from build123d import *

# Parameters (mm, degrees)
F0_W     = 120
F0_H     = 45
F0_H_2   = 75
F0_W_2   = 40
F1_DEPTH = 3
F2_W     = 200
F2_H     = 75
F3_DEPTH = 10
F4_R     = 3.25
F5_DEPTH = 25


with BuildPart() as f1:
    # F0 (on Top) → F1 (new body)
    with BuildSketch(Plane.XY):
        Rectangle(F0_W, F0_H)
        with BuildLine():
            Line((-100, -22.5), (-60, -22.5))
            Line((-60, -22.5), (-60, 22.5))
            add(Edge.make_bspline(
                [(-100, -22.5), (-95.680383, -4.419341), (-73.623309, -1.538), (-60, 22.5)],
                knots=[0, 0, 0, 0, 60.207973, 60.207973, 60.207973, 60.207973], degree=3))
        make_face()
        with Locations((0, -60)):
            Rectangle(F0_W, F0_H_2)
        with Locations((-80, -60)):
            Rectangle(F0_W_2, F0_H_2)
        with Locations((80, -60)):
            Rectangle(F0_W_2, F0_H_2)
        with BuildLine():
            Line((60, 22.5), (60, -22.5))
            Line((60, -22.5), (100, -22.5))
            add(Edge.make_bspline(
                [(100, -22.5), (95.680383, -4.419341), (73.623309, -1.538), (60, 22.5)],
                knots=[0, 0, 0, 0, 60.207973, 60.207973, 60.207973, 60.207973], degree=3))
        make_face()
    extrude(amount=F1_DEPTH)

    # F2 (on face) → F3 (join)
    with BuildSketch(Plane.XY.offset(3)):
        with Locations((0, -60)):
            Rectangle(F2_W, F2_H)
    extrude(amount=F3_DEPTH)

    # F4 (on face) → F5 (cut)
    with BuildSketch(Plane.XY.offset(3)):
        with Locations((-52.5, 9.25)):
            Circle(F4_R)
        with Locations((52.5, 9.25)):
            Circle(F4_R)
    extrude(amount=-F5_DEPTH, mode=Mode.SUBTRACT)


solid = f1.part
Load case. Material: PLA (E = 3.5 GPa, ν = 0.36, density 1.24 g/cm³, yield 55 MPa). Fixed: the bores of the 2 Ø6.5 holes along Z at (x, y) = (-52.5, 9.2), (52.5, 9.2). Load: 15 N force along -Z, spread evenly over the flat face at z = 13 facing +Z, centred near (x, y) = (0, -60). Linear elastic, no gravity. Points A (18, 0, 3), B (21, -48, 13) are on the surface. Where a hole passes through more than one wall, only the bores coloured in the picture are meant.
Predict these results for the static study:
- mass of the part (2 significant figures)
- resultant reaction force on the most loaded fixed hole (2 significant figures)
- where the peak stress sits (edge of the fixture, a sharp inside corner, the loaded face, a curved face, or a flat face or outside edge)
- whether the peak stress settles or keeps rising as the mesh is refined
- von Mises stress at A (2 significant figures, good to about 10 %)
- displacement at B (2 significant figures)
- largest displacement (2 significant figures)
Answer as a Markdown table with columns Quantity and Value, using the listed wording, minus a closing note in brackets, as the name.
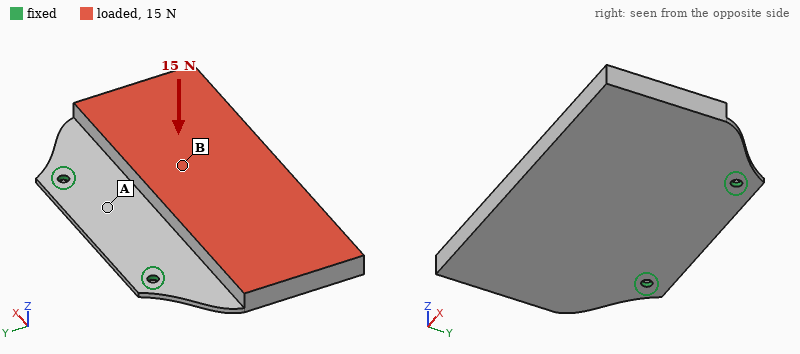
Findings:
| Quantity | Value |
|---|---|
| mass of the part | 270 g |
| resultant reaction force on the most loaded fixed hole | 7.5 N |
| where the peak stress sits | edge of the fixture |
| whether the peak stress settles or keeps rising as the mesh is refined | keeps rising |
| von Mises stress at A | 1.9 MPa |
| displacement at B | 1.2 mm |
| largest displacement | 2.4 mm |
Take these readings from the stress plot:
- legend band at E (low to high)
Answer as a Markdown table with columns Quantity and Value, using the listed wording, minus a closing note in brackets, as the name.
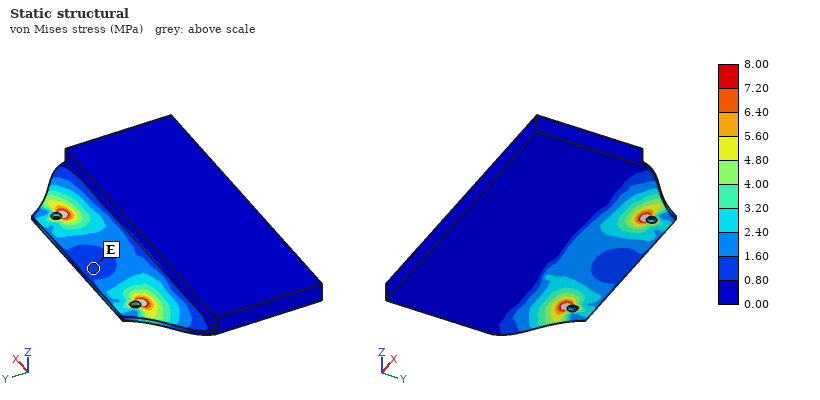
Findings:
| Quantity | Value |
|---|---|
| legend band at E | 0.80 to 1.60 MPa |
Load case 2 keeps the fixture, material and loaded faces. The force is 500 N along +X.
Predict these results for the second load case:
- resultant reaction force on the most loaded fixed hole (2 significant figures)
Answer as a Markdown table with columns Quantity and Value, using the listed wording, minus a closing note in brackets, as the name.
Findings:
| Quantity | Value |
|---|---|
| resultant reaction force on the most loaded fixed hole | 410 N |
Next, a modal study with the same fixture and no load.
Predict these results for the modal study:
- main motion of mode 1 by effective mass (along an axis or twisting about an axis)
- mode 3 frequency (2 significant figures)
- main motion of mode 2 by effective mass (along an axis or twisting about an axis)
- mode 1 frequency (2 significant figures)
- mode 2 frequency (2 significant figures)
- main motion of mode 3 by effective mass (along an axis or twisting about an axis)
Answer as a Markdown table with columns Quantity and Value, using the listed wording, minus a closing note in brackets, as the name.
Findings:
| Quantity | Value |
|---|---|
| main motion of mode 1 by effective mass | along Z |
| mode 3 frequency | 400 Hz |
| main motion of mode 2 by effective mass | twisting about Y |
| mode 1 frequency | 31 Hz |
| mode 2 frequency | 140 Hz |
| main motion of mode 3 by effective mass | along Z |
